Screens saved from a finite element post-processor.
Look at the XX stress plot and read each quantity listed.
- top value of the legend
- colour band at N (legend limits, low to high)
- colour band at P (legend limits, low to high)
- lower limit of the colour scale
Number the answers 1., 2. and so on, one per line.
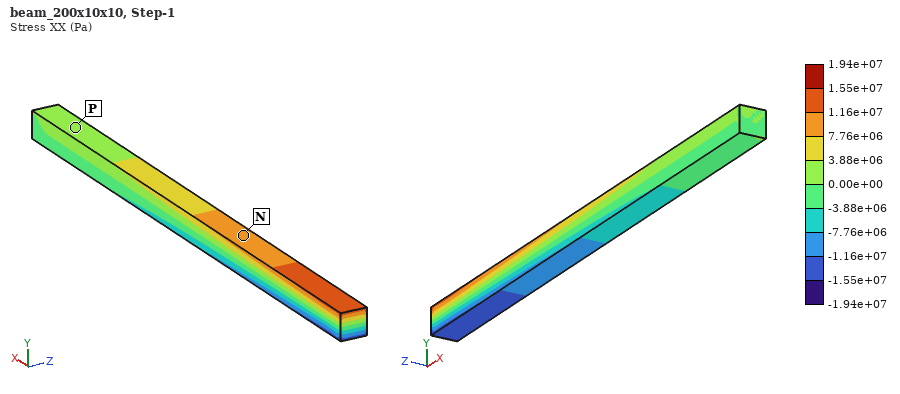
1. 1.94e+07 Pa
2. 7.76e+06 to 1.16e+07 Pa
3. 0.00e+00 to 3.88e+06 Pa
4. -1.94e+07 Pa
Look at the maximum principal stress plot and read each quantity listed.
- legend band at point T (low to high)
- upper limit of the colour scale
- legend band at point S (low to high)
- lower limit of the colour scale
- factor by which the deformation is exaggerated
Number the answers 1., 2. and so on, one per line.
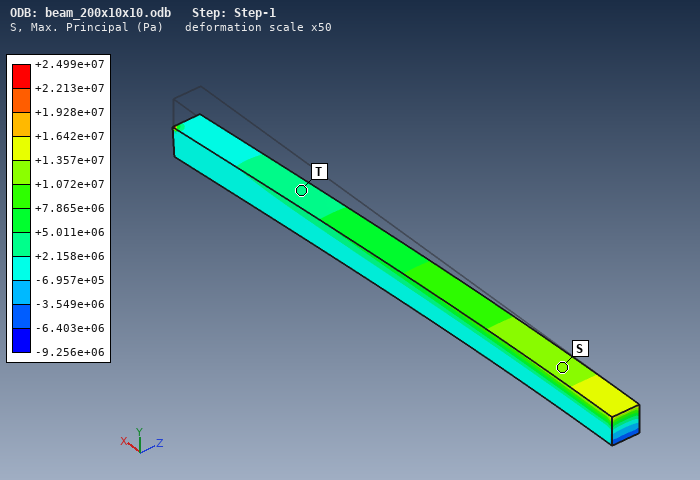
1. +2.158e+06 to +5.011e+06 Pa
2. +2.499e+07 Pa
3. +1.072e+07 to +1.357e+07 Pa
4. -9.256e+06 Pa
5. 50
